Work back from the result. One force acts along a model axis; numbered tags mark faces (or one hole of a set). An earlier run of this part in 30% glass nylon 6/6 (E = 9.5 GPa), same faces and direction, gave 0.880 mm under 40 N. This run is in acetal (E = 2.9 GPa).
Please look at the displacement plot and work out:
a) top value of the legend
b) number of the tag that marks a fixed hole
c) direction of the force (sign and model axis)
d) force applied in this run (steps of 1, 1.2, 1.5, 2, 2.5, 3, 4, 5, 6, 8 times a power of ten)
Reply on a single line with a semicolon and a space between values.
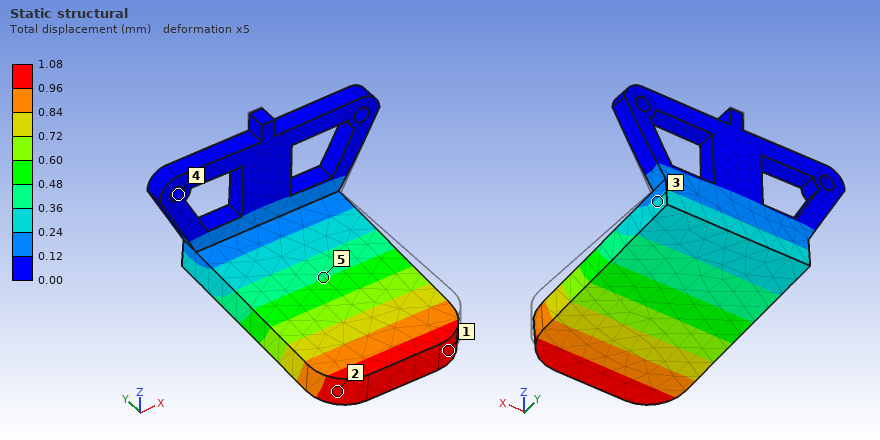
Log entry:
1.08 mm; 4; -Z; 15 N
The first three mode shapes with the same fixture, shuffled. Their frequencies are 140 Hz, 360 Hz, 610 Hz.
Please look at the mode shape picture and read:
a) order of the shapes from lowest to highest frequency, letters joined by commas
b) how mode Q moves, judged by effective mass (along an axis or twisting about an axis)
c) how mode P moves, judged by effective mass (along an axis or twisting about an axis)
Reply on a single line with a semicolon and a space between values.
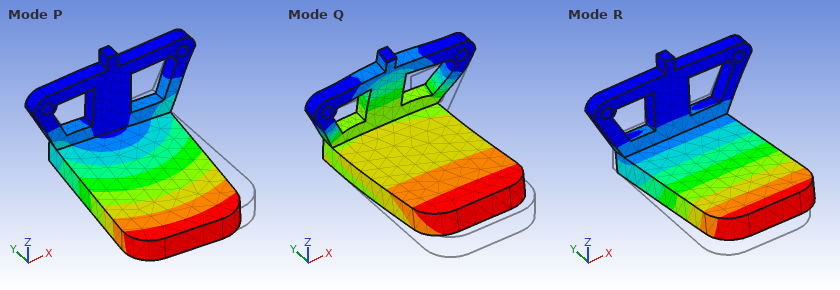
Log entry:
R, P, Q; along Y; along X
